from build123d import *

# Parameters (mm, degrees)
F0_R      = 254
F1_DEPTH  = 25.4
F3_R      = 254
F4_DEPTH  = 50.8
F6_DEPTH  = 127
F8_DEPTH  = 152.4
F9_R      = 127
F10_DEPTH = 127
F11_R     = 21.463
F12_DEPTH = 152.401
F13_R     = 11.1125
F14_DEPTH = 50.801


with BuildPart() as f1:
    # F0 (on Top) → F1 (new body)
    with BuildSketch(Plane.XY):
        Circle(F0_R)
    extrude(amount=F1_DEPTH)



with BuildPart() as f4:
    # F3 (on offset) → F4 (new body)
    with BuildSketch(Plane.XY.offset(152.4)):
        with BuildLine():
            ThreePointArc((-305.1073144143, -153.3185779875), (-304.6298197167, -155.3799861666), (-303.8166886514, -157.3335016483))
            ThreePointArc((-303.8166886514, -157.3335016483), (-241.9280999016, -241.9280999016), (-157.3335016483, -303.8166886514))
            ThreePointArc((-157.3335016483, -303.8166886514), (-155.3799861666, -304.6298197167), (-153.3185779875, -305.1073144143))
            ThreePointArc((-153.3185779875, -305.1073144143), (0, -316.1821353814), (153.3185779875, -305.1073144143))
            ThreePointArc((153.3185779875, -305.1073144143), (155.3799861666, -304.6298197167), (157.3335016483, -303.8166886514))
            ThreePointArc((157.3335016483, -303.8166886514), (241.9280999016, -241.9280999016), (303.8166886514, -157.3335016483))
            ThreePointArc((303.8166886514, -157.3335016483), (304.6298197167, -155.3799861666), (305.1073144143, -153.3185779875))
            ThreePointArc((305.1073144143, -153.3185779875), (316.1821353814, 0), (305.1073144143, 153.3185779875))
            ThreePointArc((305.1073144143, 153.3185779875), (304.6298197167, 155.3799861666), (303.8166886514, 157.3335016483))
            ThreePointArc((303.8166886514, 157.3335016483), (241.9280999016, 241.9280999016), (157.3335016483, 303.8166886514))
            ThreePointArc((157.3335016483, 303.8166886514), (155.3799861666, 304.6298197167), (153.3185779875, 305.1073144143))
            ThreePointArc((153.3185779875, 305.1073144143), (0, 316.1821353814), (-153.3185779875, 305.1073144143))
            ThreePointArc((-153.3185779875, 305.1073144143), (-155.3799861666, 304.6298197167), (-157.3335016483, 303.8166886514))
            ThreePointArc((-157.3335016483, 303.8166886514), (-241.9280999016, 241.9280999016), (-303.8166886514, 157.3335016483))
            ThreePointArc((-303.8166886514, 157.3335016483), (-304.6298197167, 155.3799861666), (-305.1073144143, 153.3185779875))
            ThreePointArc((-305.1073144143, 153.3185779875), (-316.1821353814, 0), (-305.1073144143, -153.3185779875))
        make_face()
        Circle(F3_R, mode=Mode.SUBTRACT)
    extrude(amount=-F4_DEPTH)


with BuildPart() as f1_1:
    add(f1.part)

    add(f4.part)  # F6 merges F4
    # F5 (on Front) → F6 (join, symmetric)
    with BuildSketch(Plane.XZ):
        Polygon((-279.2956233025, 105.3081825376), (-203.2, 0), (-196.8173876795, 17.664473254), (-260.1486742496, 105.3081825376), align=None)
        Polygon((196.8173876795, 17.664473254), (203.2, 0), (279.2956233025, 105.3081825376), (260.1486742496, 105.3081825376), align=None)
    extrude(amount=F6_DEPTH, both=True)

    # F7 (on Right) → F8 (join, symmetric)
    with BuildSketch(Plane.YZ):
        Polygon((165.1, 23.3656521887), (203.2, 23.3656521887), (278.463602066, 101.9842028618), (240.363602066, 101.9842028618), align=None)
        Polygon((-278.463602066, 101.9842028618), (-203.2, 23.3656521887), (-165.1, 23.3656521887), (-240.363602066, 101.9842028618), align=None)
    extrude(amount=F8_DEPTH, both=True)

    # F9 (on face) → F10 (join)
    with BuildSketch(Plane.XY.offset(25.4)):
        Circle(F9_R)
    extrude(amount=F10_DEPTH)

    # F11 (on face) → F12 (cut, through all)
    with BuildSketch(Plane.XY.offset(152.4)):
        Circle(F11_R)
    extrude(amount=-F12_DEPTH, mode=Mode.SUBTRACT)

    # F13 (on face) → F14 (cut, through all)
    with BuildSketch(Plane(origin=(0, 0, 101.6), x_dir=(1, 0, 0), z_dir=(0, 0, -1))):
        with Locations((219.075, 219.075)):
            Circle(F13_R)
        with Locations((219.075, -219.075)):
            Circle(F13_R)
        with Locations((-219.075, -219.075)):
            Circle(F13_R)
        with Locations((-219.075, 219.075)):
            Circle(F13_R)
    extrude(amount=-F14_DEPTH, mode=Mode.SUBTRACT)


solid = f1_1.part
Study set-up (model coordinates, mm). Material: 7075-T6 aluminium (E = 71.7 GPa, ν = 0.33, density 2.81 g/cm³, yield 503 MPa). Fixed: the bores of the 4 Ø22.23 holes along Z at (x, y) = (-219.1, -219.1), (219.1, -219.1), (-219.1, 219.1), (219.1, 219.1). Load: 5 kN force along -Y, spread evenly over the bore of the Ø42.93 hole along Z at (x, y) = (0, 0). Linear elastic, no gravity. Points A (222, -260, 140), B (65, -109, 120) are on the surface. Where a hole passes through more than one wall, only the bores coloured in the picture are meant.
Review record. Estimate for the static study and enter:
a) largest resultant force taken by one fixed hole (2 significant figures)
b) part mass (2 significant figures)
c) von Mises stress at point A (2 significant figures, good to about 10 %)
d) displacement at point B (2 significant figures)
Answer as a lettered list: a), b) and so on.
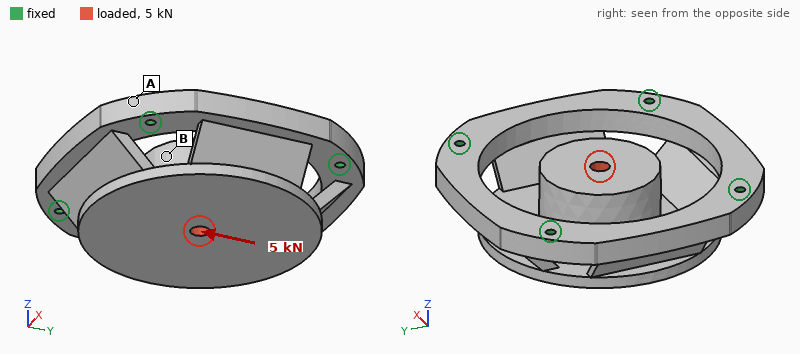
a) 1.3 kN
b) 59 kg
c) 0.41 MPa
d) 13 µm
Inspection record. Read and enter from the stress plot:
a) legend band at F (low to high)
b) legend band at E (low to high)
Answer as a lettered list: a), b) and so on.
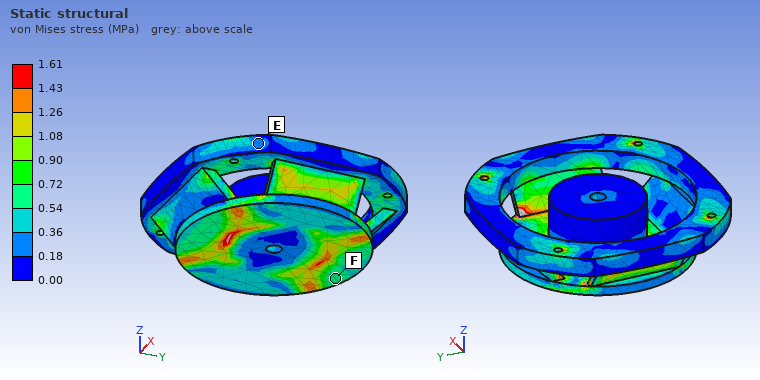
a) 0.54 to 0.72 MPa
b) 0.18 to 0.36 MPa
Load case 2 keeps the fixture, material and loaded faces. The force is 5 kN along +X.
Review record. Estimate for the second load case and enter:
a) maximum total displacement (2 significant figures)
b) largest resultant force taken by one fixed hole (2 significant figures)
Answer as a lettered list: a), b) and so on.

a) 12 µm
b) 1.3 kN
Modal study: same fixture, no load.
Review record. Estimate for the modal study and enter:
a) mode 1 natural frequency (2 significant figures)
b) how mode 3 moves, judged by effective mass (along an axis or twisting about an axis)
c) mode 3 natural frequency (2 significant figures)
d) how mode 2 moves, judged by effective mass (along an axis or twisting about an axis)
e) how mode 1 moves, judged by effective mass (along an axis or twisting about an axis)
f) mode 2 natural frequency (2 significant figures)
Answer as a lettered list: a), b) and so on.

a) 620 Hz
b) along X
c) 750 Hz
d) along Y
e) along Z
f) 650 Hz
